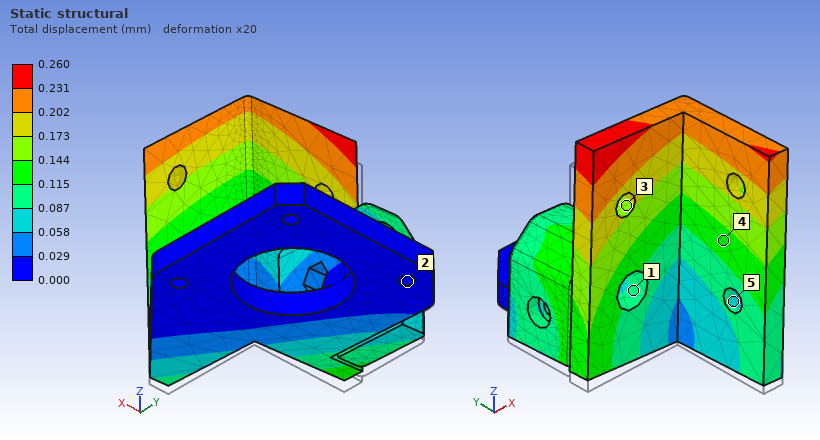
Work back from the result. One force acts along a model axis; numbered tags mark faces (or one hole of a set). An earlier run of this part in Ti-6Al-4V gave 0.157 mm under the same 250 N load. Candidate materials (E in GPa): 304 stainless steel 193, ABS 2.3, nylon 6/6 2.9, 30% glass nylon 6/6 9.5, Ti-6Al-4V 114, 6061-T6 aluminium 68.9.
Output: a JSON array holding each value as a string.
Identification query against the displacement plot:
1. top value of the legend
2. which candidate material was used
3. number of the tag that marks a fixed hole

["0.260 mm", "6061-T6 aluminium", "2"]
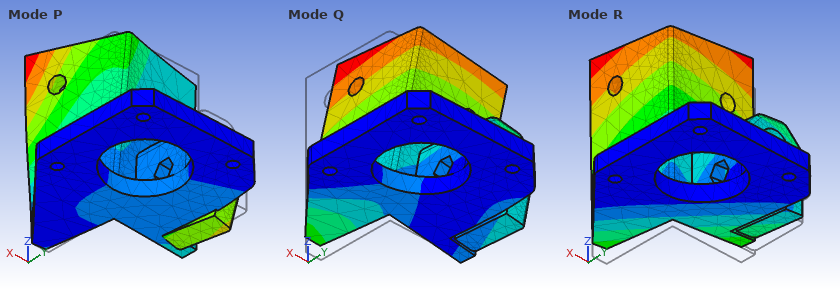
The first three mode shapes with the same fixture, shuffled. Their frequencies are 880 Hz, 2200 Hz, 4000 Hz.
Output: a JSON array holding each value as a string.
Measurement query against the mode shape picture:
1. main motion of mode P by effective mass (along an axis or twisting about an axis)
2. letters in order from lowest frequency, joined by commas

["along Z", "R, Q, P"]
